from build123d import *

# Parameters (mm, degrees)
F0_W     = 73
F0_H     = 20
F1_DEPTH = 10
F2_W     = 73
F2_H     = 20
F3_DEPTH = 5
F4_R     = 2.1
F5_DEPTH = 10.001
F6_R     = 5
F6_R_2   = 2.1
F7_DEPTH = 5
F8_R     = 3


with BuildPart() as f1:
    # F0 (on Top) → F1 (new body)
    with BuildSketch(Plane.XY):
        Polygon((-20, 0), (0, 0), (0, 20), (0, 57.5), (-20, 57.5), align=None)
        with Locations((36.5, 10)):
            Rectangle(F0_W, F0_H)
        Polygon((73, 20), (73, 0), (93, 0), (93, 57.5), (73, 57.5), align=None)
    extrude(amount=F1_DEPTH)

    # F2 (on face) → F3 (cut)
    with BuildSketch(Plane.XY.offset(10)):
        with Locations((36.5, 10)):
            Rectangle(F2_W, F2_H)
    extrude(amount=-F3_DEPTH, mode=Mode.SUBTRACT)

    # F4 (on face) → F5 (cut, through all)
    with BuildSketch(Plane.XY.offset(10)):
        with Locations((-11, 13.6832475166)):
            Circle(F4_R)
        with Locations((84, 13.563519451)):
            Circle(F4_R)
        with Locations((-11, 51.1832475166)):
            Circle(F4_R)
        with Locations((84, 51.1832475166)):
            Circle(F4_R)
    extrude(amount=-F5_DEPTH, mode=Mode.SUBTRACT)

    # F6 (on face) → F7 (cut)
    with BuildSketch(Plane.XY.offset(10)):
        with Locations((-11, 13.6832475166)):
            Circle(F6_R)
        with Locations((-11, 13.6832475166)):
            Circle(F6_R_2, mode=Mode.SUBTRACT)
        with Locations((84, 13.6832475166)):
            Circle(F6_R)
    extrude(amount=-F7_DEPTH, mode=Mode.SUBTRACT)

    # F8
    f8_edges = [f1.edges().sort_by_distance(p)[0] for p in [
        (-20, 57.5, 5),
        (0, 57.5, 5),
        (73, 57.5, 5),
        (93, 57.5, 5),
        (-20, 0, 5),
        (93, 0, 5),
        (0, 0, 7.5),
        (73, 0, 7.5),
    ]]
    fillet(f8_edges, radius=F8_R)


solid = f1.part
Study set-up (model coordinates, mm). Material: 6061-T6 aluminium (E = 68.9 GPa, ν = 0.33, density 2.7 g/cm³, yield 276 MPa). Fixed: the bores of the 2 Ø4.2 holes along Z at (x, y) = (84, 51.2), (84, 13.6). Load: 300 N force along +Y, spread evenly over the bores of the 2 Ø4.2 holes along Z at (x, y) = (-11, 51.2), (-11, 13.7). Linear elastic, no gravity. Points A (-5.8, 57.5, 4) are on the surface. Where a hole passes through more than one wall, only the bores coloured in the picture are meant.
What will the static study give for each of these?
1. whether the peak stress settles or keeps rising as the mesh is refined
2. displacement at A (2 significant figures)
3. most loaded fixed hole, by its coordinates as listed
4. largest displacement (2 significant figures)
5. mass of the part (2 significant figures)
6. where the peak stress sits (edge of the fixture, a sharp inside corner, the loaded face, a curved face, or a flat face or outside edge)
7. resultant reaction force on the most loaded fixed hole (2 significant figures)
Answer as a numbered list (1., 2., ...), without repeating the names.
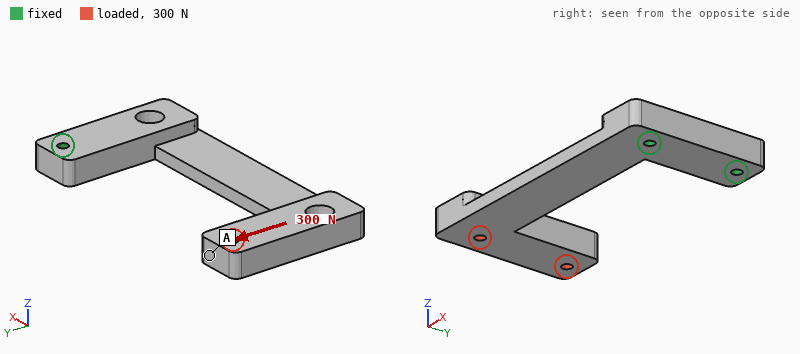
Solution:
1. keeps rising
2. 0.48 mm
3. (84, 51.2)
4. 0.56 mm
5. 78 g
6. edge of the fixture
7. 830 N
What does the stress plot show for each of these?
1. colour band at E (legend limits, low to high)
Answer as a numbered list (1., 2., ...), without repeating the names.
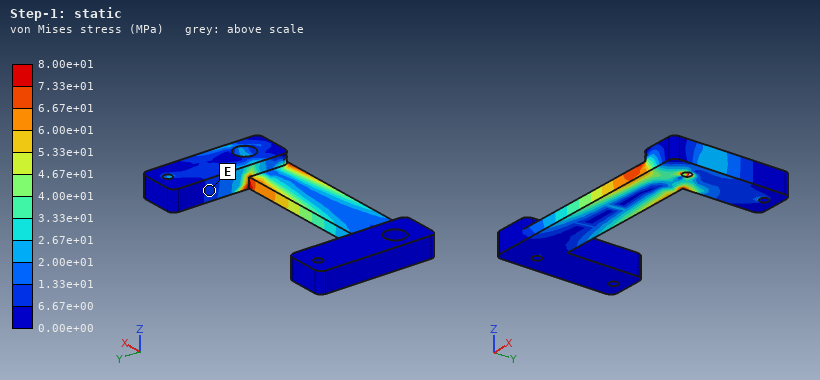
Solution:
1. 6.67e+00 to 1.33e+01 MPa
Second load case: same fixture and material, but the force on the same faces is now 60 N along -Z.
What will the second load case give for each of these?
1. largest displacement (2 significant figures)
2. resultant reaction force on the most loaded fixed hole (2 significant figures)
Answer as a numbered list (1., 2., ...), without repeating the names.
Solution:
1. 1.4 mm
2. 62 N
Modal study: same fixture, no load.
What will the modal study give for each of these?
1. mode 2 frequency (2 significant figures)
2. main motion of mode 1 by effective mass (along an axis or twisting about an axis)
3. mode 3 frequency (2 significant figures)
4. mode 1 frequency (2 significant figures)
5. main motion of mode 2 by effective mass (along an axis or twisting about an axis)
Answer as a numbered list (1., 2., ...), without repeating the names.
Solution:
1. 710 Hz
2. along Z
3. 850 Hz
4. 210 Hz
5. along Y
